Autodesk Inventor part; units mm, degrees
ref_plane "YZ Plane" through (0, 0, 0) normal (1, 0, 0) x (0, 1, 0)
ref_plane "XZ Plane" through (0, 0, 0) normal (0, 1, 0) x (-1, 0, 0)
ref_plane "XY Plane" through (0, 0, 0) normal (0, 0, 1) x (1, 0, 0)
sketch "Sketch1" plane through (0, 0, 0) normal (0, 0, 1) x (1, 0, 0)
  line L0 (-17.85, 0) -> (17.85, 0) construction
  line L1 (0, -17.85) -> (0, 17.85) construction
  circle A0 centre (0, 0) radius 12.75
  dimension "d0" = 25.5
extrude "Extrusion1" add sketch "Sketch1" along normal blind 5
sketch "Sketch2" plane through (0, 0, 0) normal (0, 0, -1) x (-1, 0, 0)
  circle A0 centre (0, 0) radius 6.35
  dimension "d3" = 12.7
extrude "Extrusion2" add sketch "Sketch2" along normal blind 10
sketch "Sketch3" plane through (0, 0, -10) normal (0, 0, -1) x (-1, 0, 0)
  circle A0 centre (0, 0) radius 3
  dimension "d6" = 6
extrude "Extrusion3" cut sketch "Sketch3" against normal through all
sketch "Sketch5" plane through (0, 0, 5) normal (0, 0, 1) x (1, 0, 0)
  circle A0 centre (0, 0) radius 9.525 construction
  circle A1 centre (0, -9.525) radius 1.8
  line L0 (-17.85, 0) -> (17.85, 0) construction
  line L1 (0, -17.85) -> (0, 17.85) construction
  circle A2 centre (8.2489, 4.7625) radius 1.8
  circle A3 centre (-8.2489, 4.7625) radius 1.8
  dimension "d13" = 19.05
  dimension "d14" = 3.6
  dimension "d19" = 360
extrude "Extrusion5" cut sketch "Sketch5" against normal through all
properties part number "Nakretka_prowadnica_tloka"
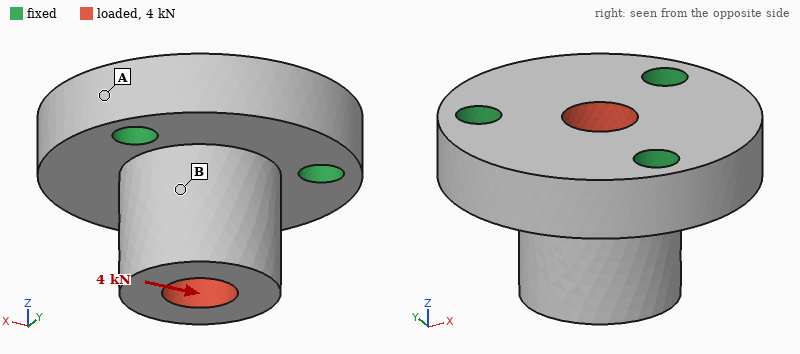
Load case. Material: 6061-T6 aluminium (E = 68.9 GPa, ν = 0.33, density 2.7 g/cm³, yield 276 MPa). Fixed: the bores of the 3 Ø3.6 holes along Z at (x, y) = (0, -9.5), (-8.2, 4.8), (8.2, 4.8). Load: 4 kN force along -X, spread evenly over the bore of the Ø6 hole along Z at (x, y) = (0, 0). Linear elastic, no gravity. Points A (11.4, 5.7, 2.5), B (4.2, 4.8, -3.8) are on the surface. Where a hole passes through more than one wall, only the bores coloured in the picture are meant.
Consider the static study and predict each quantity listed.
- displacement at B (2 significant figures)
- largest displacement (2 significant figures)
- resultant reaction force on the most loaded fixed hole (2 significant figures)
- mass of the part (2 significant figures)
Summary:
13 µm
27 µm
1.8 kN
8.8 g
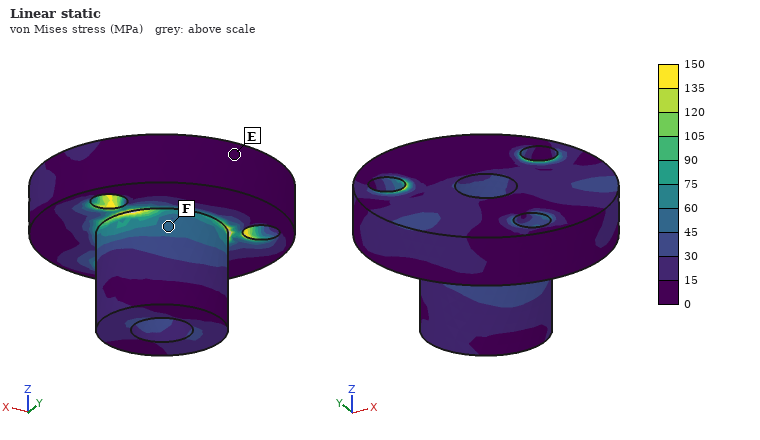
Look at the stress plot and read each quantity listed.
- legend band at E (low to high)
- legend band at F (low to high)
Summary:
0 to 15 MPa
45 to 60 MPa
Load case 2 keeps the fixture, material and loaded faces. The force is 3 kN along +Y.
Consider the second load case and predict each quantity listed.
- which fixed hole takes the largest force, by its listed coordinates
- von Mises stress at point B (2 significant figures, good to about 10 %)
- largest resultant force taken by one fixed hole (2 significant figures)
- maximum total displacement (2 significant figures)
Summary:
(0, -9.5)
22 MPa
1.5 kN
20 µm
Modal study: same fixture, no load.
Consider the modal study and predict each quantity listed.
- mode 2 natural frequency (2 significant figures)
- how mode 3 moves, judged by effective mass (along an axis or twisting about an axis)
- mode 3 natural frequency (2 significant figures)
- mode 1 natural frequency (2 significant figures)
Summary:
35 kHz
along Z
51 kHz
35 kHz
